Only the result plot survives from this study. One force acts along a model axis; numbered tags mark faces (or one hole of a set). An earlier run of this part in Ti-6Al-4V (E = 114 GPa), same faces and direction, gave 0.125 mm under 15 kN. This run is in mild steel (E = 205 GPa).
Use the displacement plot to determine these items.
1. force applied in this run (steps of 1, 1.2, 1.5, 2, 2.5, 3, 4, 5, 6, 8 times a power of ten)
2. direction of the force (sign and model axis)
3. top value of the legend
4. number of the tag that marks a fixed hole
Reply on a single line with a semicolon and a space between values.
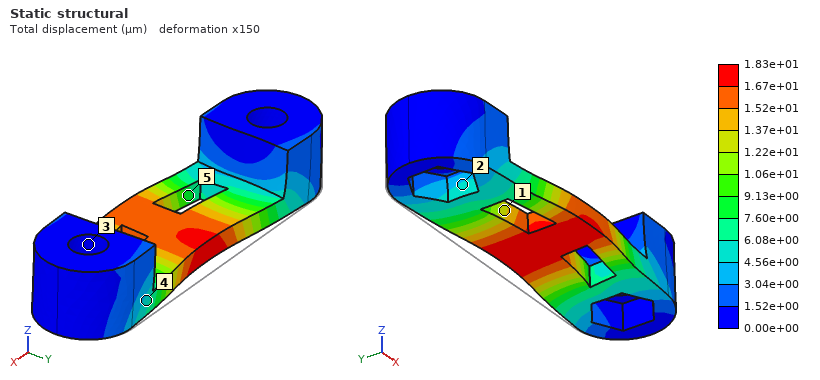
4 kN; -Y; 1.83e+01 µm; 3
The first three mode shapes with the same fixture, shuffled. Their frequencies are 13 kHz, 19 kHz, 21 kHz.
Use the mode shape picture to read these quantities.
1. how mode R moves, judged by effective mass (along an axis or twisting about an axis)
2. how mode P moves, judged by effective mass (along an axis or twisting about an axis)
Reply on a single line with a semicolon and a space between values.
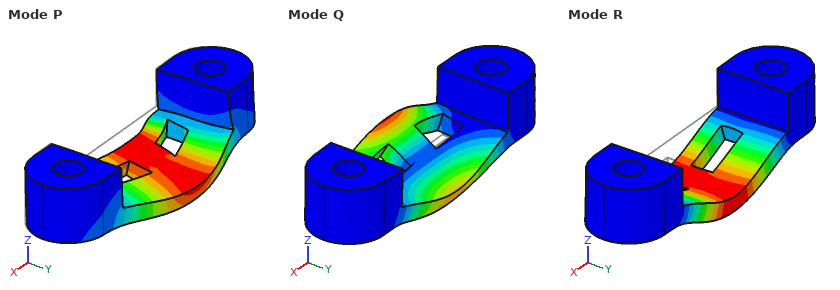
along Z; along Y
